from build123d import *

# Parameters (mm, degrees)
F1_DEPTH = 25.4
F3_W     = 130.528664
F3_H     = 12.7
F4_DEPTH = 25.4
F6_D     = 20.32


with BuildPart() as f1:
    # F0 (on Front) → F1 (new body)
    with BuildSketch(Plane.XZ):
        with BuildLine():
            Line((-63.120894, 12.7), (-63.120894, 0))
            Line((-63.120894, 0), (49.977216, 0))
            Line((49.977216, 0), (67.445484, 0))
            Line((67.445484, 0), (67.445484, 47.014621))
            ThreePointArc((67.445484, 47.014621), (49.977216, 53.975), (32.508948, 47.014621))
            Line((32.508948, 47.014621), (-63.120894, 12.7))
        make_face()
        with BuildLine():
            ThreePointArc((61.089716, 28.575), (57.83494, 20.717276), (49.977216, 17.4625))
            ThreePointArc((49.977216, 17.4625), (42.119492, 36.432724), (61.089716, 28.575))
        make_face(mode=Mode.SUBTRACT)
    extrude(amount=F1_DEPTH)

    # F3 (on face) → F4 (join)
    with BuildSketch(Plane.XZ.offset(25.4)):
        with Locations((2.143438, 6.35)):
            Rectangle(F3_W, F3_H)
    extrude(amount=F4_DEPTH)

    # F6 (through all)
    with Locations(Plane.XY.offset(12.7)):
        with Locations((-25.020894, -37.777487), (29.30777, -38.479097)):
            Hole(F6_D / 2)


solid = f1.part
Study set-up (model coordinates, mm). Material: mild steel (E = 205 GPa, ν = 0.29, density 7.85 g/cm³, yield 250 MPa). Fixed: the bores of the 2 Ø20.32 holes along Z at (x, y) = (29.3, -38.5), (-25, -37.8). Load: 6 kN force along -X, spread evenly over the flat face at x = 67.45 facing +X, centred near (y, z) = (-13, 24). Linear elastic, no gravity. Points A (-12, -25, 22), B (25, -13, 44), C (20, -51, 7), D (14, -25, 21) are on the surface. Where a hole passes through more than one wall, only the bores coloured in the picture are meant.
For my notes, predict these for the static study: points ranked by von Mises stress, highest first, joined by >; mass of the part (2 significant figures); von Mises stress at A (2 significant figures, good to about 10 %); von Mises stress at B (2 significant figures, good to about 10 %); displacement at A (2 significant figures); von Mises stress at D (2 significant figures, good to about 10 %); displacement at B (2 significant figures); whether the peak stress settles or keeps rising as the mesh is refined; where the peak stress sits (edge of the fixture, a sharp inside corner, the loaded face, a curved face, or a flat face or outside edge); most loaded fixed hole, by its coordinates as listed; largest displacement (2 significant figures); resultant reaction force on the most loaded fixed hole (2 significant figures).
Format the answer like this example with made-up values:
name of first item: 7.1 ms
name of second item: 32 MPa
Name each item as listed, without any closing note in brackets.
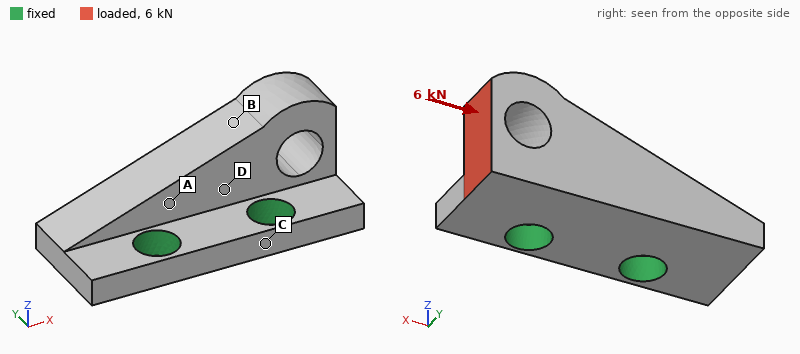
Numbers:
points ranked by von Mises stress, highest first, joined by >: B > A > D > C
mass of the part: 1.1 kg
von Mises stress at A: 8.2 MPa
von Mises stress at B: 12 MPa
displacement at A: 1.5 µm
von Mises stress at D: 5.9 MPa
displacement at B: 4.1 µm
whether the peak stress settles or keeps rising as the mesh is refined: keeps rising
where the peak stress sits: edge of the fixture
most loaded fixed hole, by its coordinates as listed: (29.3, -38.5)
largest displacement: 8.1 µm
resultant reaction force on the most loaded fixed hole: 4.0 kN
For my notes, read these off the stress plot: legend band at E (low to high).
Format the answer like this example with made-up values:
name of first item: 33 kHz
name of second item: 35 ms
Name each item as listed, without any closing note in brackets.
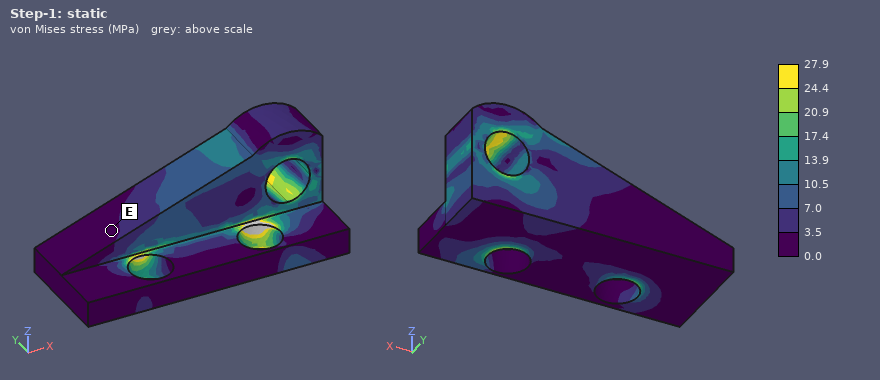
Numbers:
legend band at E: 0.0 to 3.5 MPa
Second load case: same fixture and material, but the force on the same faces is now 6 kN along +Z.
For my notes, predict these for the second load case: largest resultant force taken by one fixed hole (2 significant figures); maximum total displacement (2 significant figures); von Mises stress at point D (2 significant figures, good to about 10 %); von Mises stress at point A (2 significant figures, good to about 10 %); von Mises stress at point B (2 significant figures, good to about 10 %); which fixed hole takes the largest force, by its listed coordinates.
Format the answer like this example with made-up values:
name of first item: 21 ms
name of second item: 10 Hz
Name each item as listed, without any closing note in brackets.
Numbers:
largest resultant force taken by one fixed hole: 8.6 kN
maximum total displacement: 41 µm
von Mises stress at point D: 20 MPa
von Mises stress at point A: 22 MPa
von Mises stress at point B: 24 MPa
which fixed hole takes the largest force, by its listed coordinates: (29.3, -38.5)
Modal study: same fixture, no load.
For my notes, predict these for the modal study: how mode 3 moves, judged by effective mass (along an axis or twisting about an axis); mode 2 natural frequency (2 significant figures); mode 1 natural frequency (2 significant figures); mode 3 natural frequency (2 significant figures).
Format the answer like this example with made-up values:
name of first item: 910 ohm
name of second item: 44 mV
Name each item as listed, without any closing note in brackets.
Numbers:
how mode 3 moves, judged by effective mass: along Z
mode 2 natural frequency: 6200 Hz
mode 1 natural frequency: 3400 Hz
mode 3 natural frequency: 8200 Hz
